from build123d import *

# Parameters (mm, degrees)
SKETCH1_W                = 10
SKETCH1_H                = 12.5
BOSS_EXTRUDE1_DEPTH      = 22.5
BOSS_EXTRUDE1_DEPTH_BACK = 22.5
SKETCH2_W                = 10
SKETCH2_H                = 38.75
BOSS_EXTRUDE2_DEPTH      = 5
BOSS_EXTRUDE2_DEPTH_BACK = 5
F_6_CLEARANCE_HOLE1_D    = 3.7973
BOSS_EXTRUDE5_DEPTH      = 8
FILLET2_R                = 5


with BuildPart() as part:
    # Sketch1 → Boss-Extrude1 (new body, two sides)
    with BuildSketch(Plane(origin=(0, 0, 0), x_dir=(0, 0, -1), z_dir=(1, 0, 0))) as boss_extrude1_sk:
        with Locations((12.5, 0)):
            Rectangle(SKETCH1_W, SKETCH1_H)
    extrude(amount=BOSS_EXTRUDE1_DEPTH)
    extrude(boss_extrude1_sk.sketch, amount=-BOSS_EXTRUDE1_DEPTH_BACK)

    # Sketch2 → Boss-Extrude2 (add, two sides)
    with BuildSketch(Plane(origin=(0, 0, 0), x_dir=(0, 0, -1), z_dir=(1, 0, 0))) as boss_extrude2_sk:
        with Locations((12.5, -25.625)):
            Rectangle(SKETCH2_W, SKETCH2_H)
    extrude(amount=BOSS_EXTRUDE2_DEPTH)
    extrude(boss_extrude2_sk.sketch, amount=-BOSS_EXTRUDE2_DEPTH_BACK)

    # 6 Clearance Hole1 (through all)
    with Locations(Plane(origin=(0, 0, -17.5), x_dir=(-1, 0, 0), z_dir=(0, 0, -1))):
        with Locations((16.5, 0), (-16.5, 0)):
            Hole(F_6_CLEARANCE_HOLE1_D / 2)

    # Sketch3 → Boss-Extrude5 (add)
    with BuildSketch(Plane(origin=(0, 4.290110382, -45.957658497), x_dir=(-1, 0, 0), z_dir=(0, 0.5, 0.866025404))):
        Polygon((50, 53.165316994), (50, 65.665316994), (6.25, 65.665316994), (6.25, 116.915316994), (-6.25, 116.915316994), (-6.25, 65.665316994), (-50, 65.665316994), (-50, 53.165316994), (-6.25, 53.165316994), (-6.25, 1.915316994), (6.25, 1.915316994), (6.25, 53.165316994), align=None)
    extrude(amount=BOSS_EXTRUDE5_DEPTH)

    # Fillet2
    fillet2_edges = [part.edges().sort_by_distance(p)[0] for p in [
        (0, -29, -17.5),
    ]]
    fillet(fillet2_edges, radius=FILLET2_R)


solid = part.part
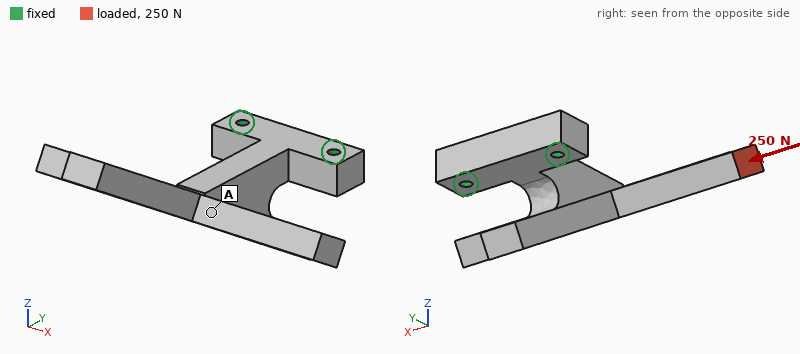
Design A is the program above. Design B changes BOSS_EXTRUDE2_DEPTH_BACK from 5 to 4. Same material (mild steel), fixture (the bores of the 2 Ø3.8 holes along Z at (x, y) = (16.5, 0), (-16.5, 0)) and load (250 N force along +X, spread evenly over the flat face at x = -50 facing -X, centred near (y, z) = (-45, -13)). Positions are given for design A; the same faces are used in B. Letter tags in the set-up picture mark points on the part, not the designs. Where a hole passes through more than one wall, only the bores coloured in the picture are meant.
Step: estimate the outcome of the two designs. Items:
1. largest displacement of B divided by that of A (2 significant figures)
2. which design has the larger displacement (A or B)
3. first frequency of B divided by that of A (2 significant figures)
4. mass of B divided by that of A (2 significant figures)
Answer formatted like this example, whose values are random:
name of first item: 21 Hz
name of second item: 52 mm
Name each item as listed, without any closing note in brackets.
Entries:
largest displacement of B divided by that of A: 1.3
which design has the larger displacement: B
first frequency of B divided by that of A: 0.91
mass of B divided by that of A: 0.99
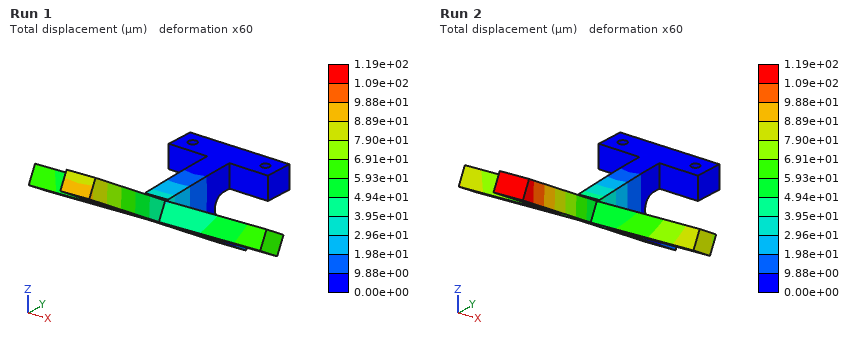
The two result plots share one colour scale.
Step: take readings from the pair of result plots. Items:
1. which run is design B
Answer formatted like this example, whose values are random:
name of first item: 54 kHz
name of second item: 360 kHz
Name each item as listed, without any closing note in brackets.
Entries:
which run is design B: Run 2
